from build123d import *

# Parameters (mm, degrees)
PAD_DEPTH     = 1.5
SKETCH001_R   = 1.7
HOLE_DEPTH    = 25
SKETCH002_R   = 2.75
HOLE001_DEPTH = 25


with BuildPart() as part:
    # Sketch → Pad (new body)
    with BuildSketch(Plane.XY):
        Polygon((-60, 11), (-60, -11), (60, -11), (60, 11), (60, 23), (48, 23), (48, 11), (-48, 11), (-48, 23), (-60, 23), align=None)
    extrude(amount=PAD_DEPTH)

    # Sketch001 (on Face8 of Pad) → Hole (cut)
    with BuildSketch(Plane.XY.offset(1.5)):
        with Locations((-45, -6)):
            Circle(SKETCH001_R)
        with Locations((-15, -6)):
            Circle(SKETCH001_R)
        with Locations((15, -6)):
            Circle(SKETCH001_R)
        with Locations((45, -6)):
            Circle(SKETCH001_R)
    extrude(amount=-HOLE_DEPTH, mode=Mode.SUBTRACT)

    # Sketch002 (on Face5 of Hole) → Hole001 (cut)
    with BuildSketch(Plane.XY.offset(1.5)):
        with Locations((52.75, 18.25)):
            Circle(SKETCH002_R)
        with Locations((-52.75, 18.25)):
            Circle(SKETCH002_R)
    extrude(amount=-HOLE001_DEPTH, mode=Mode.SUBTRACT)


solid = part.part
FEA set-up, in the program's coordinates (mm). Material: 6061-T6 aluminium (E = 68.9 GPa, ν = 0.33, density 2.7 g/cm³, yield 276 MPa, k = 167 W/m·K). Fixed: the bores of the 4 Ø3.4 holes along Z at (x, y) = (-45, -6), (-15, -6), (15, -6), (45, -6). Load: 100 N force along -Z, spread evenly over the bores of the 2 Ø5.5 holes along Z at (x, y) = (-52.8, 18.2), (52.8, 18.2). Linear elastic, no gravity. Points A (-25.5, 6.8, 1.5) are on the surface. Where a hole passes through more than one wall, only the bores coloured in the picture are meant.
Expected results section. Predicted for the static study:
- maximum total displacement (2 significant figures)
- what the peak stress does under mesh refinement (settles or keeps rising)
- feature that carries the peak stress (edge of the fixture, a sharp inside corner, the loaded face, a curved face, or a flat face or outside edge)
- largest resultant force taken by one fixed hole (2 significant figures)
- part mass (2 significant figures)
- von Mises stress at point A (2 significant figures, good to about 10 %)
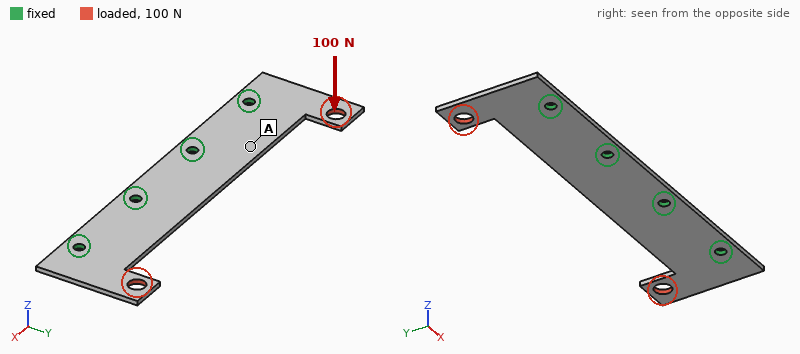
0.87 mm
keeps rising
edge of the fixture
57 N
12 g
25 MPa
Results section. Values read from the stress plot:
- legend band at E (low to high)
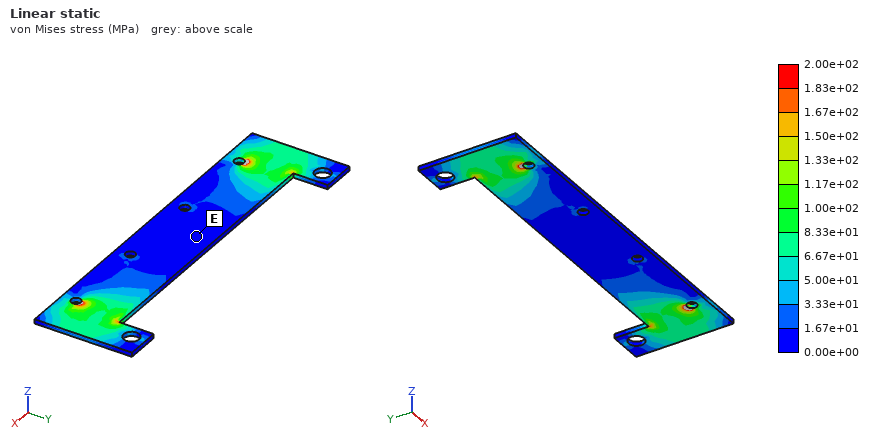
0.00e+00 to 1.67e+01 MPa
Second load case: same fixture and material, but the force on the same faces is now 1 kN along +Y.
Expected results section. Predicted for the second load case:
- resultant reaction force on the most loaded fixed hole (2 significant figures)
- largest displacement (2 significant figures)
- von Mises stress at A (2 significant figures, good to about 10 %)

590 N
27 µm
9.5 MPa
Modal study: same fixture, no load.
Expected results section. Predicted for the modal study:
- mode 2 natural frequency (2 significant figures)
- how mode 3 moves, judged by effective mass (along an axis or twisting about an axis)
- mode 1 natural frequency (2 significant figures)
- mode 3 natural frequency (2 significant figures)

1900 Hz
along Z
1900 Hz
3800 Hz
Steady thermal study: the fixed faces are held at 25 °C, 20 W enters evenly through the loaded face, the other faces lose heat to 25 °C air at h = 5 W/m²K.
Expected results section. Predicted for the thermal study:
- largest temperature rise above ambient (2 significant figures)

80 K
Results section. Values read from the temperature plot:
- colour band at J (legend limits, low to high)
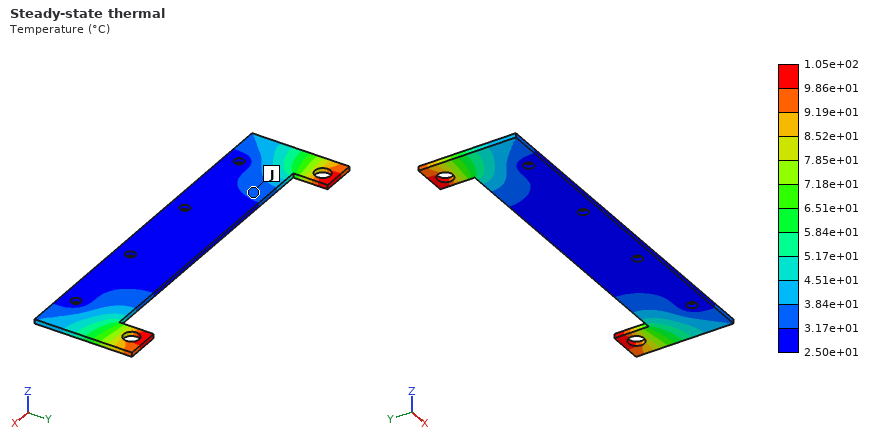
3.17e+01 to 3.84e+01 °C
